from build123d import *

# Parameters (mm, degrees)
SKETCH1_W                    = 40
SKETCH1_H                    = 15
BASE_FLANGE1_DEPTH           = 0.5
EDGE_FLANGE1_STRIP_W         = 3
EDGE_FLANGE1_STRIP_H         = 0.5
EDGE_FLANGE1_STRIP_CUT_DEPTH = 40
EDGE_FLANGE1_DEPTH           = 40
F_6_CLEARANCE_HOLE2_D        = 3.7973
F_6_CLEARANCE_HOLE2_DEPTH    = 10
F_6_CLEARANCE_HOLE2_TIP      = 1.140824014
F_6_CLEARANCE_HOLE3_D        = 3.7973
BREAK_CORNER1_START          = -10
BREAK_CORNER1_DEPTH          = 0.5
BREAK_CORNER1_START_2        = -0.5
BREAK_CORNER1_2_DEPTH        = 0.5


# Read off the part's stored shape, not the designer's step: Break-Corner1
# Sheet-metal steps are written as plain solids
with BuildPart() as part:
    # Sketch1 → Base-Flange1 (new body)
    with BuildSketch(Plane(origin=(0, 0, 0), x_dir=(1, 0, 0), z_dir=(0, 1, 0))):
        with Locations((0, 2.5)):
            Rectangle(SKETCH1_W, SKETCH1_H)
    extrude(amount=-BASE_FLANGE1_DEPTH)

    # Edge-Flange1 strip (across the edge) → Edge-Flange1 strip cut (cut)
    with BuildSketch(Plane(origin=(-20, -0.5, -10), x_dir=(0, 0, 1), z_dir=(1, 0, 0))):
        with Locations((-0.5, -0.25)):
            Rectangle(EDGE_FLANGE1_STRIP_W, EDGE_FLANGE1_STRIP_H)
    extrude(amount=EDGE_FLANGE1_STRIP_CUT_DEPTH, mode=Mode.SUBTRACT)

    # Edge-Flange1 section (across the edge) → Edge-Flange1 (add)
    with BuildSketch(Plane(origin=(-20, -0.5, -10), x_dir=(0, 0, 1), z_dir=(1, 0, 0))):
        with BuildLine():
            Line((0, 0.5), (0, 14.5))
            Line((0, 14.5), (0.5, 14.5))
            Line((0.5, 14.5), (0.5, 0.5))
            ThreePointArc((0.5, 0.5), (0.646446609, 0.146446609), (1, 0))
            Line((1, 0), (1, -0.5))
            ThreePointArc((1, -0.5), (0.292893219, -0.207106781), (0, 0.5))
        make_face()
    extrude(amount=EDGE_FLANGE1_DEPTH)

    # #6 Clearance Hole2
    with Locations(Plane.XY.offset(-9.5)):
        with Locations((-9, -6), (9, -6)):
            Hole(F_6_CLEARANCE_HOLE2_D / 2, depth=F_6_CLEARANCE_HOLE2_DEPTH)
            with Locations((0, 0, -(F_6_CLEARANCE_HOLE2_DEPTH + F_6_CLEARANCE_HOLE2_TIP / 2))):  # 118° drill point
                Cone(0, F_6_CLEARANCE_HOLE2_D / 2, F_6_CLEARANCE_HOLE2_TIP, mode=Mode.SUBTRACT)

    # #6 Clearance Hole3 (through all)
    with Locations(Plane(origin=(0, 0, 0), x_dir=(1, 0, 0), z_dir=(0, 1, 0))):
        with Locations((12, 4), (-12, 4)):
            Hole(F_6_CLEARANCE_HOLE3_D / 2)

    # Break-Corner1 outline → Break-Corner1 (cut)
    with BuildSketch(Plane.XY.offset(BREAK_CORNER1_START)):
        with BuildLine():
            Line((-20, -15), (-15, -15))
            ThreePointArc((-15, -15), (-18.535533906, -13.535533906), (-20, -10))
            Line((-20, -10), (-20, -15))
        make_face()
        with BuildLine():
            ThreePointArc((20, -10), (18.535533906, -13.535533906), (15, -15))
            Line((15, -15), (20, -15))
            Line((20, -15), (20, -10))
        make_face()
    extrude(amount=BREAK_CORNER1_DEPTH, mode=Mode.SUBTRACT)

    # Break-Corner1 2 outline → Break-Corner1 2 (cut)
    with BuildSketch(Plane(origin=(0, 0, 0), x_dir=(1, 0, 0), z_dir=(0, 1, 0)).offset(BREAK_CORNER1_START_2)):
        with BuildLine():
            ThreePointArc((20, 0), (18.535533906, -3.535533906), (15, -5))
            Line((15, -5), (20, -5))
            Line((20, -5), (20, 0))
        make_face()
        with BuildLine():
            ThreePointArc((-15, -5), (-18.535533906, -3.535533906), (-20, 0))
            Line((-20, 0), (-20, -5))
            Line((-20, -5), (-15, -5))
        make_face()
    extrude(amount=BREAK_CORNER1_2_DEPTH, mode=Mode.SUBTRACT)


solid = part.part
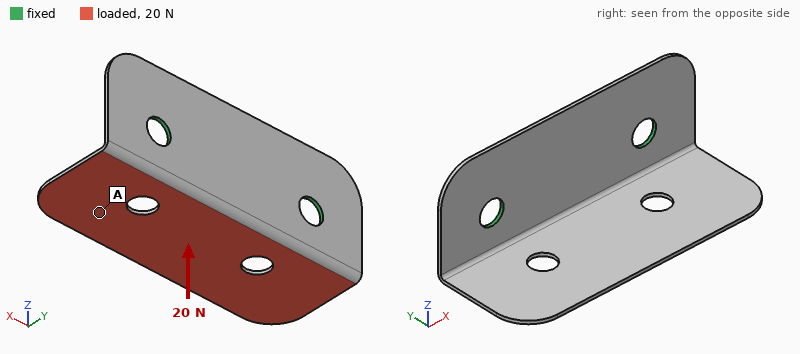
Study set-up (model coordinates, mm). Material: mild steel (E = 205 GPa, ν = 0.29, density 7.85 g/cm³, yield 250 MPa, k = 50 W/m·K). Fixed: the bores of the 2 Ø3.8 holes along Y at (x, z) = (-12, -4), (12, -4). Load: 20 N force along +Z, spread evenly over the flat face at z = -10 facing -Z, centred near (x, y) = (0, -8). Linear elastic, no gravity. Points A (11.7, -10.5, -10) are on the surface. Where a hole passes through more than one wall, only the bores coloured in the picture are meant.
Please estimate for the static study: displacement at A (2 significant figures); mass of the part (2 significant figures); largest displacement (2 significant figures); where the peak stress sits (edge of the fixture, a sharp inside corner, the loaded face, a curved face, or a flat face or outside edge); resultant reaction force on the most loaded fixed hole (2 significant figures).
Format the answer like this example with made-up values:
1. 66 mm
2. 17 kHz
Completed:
1. 0.14 mm
2. 4.3 g
3. 0.22 mm
4. a flat face or outside edge
5. 10 N
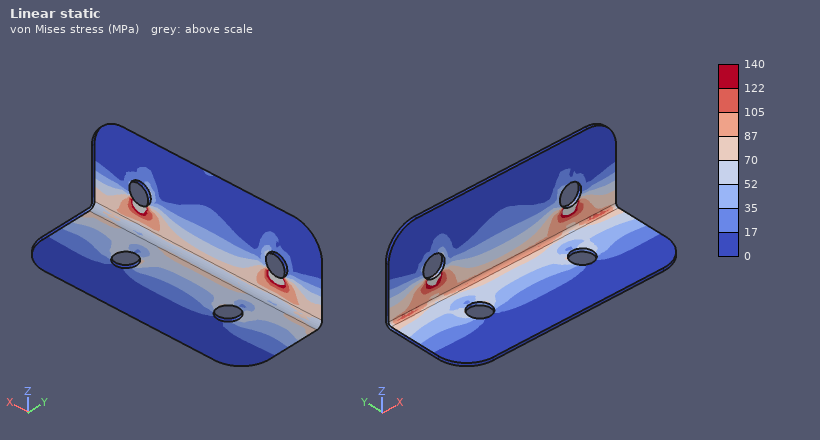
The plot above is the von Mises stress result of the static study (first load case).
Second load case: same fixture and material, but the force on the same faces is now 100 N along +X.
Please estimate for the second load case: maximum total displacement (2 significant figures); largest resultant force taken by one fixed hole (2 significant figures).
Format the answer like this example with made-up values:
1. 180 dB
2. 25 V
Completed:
1. 79 µm
2. 62 N
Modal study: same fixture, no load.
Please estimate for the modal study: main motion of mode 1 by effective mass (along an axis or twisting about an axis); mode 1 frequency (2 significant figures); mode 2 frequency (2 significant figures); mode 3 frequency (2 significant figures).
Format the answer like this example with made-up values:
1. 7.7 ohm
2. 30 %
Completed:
1. along Z
2. 1300 Hz
3. 2000 Hz
4. 3900 Hz
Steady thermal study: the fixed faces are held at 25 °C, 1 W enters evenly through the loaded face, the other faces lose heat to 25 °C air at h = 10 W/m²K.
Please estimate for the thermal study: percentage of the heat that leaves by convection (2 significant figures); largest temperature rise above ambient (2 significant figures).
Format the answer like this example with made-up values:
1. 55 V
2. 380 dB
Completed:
1. 10 %
2. 15 K
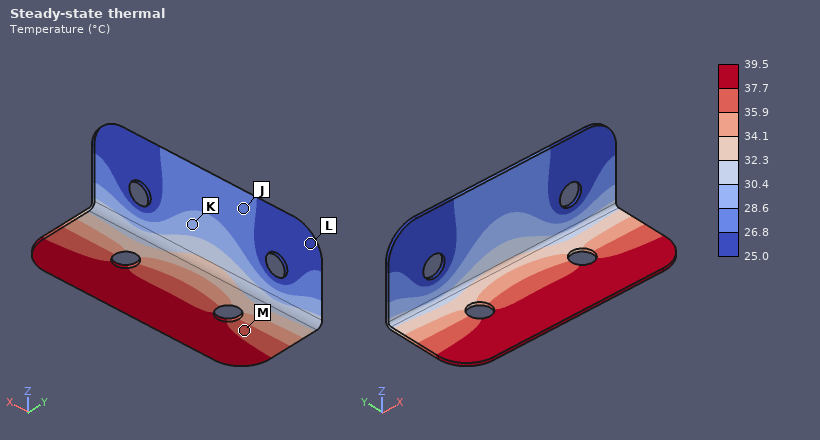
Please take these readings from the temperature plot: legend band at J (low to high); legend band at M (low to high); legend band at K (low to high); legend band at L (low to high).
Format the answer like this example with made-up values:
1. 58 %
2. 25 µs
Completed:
1. 26.8 to 28.6 °C
2. 35.9 to 37.7 °C
3. 28.6 to 30.4 °C
4. 25.0 to 26.8 °C
